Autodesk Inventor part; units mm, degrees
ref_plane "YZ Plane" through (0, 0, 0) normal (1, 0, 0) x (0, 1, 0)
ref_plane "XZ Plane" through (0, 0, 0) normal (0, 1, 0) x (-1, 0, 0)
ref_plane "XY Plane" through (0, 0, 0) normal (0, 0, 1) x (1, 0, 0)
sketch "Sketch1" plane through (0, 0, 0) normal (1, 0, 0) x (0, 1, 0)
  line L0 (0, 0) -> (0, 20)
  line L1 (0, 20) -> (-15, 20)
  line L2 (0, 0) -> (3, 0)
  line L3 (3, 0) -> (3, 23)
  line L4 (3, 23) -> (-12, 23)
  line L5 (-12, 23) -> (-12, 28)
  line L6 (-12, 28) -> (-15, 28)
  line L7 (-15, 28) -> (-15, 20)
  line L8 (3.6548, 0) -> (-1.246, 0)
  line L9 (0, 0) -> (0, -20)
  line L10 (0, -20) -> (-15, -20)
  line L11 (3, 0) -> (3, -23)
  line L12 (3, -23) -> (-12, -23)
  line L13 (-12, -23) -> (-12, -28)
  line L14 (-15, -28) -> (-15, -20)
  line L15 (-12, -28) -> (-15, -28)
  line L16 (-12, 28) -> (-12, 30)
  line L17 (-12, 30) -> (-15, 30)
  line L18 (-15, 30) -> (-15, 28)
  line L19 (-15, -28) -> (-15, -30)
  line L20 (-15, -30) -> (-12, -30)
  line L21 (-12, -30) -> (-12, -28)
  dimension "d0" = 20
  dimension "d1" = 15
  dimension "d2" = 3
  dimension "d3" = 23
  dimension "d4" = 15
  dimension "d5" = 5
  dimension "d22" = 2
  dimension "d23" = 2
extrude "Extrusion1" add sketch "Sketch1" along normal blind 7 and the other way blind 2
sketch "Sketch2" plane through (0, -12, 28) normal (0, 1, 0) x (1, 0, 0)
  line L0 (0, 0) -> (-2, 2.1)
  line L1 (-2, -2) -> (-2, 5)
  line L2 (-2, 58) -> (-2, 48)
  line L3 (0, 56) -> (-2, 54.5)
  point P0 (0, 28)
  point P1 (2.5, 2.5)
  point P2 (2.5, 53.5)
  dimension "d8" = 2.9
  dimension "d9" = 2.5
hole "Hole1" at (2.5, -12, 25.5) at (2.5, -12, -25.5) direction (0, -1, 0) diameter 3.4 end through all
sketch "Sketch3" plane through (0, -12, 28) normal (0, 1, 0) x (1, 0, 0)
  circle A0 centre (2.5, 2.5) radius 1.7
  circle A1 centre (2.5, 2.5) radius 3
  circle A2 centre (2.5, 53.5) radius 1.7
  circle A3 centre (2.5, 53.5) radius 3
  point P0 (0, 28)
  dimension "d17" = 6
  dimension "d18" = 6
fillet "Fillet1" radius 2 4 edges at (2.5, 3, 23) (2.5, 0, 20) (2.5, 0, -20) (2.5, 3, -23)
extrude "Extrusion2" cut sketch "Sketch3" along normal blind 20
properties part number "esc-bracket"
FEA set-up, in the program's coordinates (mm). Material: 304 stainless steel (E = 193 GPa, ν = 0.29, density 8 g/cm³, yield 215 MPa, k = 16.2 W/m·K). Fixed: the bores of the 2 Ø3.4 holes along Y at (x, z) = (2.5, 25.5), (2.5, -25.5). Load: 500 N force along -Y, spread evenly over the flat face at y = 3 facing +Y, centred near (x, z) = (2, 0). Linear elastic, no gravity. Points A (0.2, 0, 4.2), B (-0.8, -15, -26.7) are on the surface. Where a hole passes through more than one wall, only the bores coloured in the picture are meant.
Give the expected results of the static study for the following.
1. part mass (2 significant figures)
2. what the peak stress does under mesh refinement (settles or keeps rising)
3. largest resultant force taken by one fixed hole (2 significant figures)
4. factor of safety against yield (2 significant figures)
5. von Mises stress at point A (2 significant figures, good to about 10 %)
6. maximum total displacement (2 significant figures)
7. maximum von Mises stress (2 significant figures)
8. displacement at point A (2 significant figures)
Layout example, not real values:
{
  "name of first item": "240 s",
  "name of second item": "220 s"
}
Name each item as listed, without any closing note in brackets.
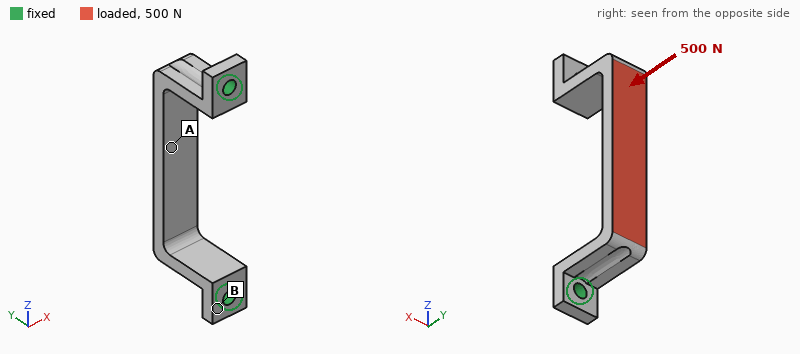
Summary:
{
  "part mass": "19 g",
  "what the peak stress does under mesh refinement": "settles",
  "largest resultant force taken by one fixed hole": "300 N",
  "factor of safety against yield": "1.7",
  "von Mises stress at point A": "64 MPa",
  "maximum total displacement": "37 µm",
  "maximum von Mises stress": "130 MPa",
  "displacement at point A": "34 µm"
}
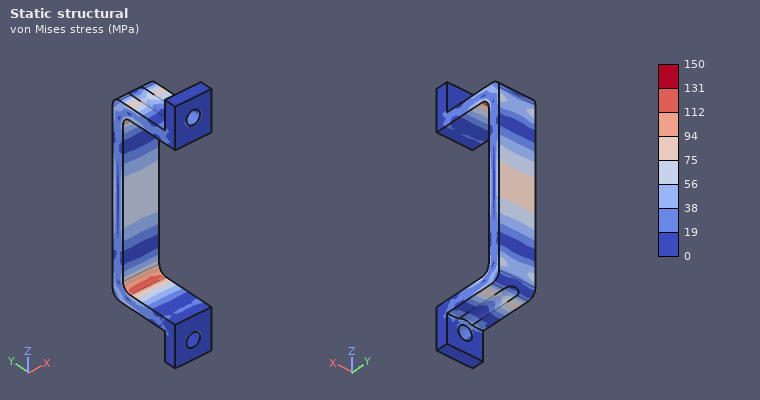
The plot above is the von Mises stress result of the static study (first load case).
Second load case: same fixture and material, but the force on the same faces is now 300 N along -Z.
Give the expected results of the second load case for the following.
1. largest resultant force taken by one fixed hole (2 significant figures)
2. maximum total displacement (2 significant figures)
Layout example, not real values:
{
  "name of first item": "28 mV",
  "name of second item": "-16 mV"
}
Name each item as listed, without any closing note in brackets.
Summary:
{
  "largest resultant force taken by one fixed hole": "160 N",
  "maximum total displacement": "27 µm"
}
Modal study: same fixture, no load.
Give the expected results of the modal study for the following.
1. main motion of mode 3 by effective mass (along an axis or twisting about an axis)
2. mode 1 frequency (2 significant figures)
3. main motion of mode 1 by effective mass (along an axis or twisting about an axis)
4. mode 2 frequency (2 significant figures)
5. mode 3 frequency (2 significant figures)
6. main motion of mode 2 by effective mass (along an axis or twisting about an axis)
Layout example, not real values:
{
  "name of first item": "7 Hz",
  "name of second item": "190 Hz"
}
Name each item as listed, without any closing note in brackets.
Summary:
{
  "main motion of mode 3 by effective mass": "along Y",
  "mode 1 frequency": "5000 Hz",
  "main motion of mode 1 by effective mass": "along Z",
  "mode 2 frequency": "5400 Hz",
  "mode 3 frequency": "7000 Hz",
  "main motion of mode 2 by effective mass": "along X"
}
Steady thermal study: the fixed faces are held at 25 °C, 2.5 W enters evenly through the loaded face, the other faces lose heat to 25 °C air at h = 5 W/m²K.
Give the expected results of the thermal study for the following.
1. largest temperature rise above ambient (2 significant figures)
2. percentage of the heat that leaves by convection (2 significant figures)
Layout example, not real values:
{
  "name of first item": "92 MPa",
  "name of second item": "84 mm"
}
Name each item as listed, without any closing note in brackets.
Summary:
{
  "largest temperature rise above ambient": "69 K",
  "percentage of the heat that leaves by convection": "11 %"
}
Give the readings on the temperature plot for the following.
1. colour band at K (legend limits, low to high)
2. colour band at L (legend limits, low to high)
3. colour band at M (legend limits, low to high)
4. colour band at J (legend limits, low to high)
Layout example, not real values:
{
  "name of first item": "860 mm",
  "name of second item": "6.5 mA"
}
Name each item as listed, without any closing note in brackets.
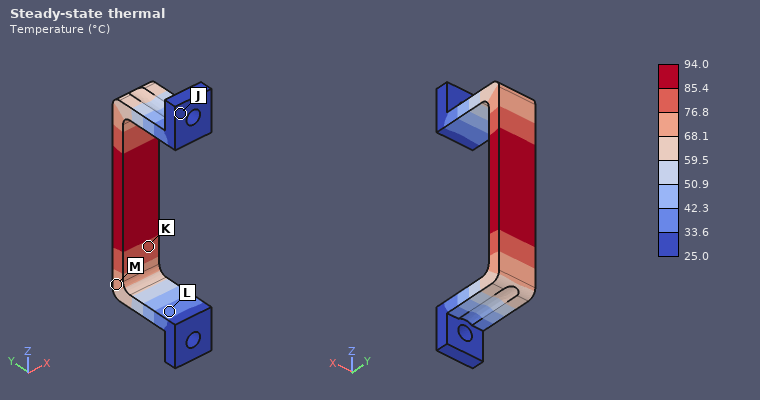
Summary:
{
  "colour band at K": "76.8 to 85.4 °C",
  "colour band at L": "33.6 to 42.3 °C",
  "colour band at M": "68.1 to 76.8 °C",
  "colour band at J": "25.0 to 33.6 °C"
}
